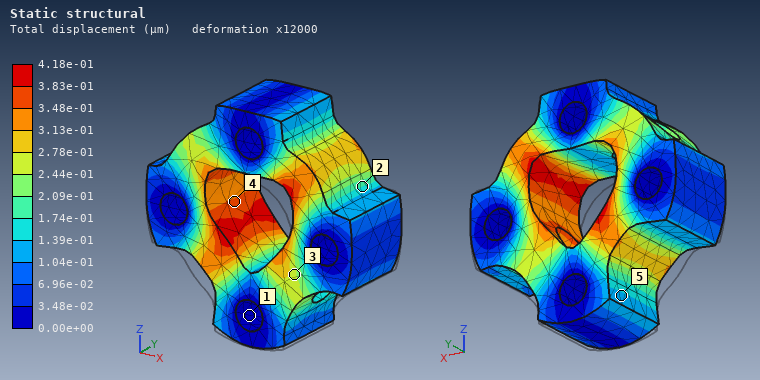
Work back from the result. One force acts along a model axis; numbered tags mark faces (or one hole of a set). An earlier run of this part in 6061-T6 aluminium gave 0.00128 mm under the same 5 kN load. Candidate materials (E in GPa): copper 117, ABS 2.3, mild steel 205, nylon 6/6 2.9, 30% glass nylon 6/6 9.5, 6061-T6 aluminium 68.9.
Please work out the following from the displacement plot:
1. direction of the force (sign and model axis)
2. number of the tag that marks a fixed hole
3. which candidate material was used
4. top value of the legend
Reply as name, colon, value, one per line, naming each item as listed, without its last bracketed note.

direction of the force: +Z
number of the tag that marks a fixed hole: 1
which candidate material was used: mild steel
top value of the legend: 4.18e-01 µm
